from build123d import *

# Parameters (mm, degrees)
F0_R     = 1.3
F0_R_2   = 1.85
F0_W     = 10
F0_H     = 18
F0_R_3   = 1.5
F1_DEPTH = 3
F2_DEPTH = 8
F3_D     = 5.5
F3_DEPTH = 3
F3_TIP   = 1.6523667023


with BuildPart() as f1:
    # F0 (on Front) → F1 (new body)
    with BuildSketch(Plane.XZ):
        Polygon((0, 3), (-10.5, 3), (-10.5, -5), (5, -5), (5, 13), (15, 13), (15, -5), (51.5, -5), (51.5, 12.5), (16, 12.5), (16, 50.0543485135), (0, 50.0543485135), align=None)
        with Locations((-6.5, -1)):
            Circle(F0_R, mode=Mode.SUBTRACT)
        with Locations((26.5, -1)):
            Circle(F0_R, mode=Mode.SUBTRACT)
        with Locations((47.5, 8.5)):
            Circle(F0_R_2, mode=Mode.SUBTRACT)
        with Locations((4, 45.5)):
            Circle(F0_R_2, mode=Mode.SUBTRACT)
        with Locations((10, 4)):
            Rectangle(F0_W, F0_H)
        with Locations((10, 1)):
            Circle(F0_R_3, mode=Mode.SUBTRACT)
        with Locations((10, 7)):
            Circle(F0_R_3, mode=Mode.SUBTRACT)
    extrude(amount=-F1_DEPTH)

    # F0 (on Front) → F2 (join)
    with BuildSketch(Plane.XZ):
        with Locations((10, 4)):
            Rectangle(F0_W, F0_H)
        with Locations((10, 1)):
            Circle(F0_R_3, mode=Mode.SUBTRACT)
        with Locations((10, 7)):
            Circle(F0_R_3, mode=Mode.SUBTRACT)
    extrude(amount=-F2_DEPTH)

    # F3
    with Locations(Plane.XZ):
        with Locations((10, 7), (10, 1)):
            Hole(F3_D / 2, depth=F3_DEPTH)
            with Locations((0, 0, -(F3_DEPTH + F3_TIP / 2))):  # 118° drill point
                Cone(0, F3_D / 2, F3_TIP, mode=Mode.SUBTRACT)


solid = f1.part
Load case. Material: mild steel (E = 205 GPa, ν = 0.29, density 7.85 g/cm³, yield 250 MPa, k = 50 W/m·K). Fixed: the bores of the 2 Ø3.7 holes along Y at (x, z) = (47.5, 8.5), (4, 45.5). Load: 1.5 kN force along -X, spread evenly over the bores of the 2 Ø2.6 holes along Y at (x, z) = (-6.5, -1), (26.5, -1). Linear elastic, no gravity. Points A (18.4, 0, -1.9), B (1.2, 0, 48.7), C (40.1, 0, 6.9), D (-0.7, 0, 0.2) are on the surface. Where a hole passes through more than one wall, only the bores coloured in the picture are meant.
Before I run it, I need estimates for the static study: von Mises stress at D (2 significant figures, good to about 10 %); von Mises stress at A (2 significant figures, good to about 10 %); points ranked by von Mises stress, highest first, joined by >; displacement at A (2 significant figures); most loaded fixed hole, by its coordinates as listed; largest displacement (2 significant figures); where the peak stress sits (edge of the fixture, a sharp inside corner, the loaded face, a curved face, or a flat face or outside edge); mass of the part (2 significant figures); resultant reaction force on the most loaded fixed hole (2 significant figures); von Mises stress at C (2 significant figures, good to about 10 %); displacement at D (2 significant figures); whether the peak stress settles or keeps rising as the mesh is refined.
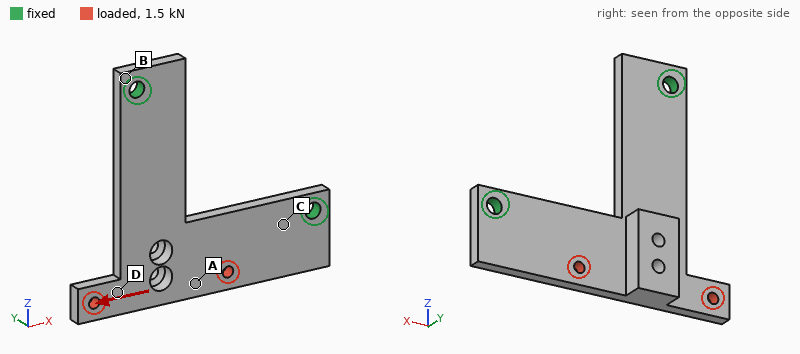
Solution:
28 MPa
20 MPa
C > D > A > B
5.6 µm
(47.5, 8.5)
13 µm
edge of the fixture
42 g
1.5 kN
44 MPa
9.5 µm
keeps rising
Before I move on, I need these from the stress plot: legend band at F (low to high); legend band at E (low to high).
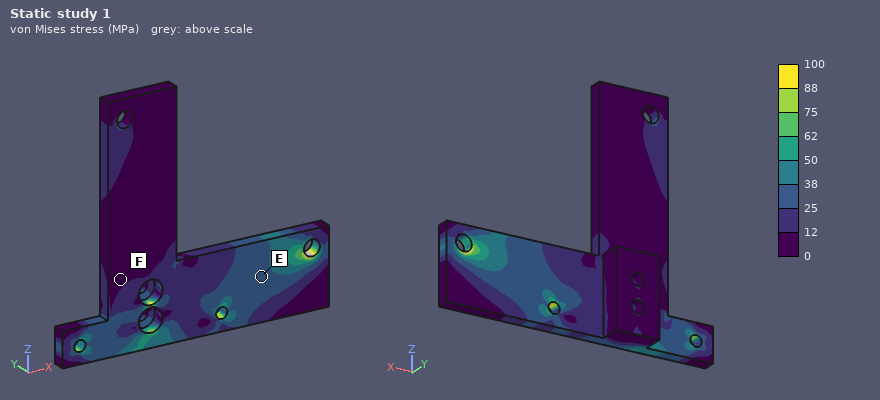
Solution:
0 to 12 MPa
25 to 38 MPa
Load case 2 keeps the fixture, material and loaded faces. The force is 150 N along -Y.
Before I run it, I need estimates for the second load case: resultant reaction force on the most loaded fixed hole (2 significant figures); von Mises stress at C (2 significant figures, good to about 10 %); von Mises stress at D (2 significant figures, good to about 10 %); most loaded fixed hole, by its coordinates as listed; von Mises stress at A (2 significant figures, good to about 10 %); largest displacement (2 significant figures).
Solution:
96 N
81 MPa
36 MPa
(47.5, 8.5)
26 MPa
0.25 mm
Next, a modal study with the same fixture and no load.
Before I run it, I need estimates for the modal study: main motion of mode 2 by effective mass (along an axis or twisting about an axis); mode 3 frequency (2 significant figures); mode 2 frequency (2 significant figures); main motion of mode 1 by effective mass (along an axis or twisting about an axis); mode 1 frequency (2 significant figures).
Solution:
along Y
5500 Hz
5100 Hz
along Y
1300 Hz
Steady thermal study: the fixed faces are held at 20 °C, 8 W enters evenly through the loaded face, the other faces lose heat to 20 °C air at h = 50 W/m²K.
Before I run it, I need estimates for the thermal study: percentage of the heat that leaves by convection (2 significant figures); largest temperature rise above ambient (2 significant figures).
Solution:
50 %
65 K
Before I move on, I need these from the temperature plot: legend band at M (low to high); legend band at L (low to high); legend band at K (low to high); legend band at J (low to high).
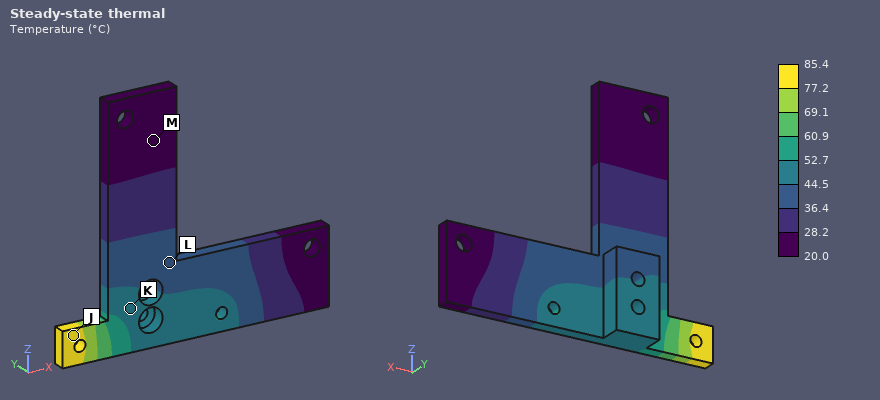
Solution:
20.0 to 28.2 °C
36.4 to 44.5 °C
44.5 to 52.7 °C
77.2 to 85.4 °C
